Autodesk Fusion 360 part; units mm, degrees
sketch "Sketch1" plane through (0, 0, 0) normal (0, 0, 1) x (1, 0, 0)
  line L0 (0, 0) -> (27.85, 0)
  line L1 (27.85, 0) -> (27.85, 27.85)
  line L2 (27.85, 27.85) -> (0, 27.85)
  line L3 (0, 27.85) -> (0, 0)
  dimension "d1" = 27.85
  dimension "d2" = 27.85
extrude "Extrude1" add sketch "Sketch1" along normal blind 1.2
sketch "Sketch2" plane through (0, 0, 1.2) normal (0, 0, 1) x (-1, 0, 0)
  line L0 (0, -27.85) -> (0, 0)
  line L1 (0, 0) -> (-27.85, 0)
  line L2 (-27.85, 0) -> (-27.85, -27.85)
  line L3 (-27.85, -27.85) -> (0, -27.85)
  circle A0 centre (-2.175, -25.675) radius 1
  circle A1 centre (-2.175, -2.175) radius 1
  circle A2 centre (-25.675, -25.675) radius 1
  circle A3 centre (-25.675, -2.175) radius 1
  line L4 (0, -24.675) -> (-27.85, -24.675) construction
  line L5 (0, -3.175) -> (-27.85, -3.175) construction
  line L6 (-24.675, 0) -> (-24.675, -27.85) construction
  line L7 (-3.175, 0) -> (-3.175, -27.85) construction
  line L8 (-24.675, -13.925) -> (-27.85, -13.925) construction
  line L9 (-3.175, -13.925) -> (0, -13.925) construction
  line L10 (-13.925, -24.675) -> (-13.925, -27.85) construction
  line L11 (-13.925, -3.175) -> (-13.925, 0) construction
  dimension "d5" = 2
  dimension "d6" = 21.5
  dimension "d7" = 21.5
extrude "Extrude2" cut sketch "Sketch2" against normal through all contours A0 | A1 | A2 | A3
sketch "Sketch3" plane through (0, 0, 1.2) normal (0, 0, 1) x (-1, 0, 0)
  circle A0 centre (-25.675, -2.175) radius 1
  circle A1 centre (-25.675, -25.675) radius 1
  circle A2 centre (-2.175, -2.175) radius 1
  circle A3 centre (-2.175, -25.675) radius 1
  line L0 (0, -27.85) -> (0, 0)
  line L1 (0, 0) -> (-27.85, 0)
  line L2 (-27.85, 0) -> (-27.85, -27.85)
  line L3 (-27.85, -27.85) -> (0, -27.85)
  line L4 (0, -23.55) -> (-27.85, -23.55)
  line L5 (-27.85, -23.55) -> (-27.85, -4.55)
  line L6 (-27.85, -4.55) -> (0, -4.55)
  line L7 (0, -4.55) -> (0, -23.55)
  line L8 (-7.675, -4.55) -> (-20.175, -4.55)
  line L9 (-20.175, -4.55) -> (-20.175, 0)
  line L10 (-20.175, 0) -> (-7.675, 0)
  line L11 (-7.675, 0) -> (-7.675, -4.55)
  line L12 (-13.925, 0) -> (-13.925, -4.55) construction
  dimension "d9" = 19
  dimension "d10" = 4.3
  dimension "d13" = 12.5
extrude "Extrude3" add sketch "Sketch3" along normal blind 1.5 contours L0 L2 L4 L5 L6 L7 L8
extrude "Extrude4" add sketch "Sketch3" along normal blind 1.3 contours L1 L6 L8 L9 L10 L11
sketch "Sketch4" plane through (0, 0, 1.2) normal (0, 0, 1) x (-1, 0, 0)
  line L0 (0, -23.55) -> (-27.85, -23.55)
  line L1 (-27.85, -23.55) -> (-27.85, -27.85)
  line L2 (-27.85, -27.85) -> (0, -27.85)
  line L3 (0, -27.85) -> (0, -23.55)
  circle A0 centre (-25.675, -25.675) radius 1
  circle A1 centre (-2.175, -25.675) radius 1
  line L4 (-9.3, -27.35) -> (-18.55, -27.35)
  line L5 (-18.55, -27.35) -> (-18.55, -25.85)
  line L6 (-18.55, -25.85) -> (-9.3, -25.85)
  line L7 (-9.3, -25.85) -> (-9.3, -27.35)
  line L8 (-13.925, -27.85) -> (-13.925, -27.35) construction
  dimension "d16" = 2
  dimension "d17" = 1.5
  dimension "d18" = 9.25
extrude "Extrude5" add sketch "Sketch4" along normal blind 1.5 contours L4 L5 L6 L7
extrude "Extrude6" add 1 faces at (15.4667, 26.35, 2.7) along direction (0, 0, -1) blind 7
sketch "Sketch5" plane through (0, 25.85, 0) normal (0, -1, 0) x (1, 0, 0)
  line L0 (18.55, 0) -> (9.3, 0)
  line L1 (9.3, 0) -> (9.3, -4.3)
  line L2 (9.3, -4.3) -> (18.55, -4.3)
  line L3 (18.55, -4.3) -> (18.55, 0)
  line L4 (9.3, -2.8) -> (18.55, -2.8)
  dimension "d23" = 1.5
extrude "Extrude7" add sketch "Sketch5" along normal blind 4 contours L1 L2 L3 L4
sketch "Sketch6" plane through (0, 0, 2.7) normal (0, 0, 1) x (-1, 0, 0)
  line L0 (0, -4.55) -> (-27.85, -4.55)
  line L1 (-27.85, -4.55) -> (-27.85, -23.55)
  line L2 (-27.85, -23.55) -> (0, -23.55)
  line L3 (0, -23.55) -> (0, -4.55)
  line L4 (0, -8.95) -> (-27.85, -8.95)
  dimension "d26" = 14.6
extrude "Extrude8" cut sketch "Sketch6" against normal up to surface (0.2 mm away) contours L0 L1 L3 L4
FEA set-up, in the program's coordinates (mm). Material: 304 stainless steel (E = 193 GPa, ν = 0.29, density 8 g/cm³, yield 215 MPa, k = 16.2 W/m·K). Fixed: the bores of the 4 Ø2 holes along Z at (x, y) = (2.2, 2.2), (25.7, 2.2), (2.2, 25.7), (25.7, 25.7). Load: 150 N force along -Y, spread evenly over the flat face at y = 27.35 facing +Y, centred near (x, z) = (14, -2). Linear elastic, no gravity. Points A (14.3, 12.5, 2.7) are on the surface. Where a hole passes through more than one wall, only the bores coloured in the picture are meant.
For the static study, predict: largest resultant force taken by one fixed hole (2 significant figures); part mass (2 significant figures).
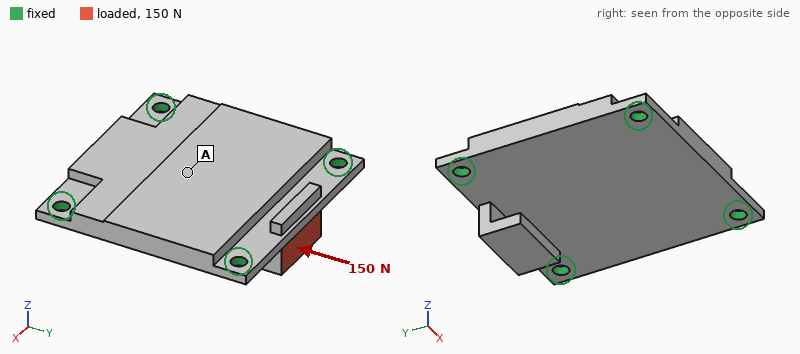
62 N
15 g
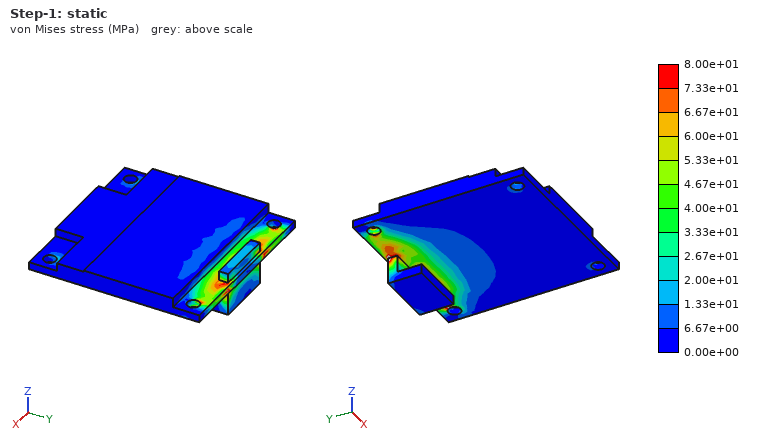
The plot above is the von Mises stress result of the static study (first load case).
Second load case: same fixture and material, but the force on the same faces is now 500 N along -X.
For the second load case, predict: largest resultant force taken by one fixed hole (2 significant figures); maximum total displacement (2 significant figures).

230 N
13 µm
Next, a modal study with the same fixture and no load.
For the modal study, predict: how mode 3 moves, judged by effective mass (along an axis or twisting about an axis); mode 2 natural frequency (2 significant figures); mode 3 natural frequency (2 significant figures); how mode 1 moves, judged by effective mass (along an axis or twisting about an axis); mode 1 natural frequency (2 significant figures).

twisting about X
13 kHz
16 kHz
along Z
11 kHz
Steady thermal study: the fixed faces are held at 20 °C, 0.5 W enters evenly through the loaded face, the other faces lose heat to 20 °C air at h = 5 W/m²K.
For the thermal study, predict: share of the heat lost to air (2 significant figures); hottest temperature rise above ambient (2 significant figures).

7.7 %
16 K
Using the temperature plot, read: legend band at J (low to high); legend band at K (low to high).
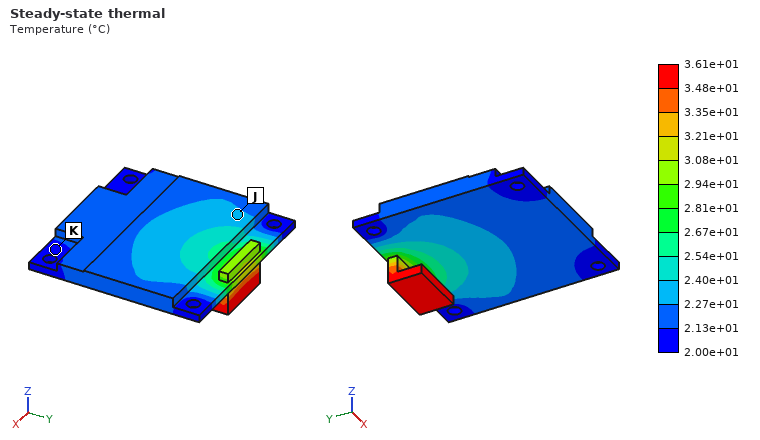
2.27e+01 to 2.40e+01 °C
2.00e+01 to 2.13e+01 °C
